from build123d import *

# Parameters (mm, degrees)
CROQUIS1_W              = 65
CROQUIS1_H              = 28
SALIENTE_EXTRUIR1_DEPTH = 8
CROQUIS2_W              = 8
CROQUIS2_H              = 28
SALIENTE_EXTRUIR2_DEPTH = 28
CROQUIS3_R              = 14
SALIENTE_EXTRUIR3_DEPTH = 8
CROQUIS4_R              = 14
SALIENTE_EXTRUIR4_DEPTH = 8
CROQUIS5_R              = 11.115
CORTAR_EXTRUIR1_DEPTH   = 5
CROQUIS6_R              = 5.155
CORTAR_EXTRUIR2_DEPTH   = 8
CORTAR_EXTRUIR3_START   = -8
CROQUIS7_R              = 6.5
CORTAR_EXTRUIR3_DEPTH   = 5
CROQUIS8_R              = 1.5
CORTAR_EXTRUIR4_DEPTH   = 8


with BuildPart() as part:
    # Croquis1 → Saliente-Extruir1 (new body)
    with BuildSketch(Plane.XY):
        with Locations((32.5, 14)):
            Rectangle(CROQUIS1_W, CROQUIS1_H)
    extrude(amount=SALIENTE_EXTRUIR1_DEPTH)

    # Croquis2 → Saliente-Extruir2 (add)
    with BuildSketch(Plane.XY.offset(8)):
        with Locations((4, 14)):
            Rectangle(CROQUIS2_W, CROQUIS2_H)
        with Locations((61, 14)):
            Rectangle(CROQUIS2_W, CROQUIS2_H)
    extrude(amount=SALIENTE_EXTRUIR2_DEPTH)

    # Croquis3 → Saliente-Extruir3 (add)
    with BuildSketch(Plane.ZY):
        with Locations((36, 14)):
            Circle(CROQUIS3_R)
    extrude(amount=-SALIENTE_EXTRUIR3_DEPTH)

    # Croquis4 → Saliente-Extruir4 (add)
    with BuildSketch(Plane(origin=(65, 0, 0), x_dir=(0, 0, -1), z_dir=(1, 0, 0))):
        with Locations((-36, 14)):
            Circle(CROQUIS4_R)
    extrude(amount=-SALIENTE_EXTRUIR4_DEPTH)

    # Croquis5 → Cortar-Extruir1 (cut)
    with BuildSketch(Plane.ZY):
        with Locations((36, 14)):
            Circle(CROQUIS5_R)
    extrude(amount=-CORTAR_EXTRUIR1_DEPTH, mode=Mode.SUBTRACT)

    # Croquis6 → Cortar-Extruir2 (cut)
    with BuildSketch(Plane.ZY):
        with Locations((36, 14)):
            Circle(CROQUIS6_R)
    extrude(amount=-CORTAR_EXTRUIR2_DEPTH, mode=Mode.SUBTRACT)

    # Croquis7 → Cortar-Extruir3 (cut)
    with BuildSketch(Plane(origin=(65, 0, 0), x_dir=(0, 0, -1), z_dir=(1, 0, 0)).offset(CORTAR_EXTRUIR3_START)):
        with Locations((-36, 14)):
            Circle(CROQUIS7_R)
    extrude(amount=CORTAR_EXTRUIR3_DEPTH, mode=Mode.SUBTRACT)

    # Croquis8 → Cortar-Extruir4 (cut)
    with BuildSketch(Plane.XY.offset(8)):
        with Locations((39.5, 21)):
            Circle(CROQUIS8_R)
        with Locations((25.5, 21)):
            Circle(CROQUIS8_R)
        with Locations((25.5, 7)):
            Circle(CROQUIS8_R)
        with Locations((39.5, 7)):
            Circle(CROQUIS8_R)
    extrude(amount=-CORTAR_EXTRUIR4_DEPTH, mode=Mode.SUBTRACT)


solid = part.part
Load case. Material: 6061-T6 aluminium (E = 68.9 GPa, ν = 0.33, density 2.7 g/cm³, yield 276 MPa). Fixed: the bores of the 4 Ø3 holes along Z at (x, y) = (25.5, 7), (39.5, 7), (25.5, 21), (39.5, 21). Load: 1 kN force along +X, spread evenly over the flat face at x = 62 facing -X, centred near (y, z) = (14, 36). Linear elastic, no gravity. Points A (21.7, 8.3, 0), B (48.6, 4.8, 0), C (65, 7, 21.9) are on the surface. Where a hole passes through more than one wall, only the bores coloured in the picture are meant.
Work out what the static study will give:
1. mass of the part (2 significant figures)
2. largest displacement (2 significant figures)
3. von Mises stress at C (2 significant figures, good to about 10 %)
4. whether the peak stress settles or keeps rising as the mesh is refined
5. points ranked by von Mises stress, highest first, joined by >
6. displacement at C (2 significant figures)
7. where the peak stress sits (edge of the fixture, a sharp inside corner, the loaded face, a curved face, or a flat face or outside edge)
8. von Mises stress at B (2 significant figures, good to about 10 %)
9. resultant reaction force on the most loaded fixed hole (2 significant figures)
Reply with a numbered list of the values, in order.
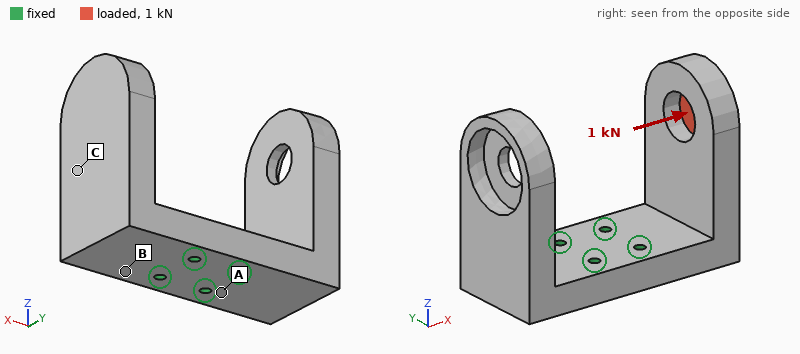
1. 78 g
2. 0.58 mm
3. 47 MPa
4. keeps rising
5. B > C > A
6. 0.23 mm
7. edge of the fixture
8. 99 MPa
9. 550 N
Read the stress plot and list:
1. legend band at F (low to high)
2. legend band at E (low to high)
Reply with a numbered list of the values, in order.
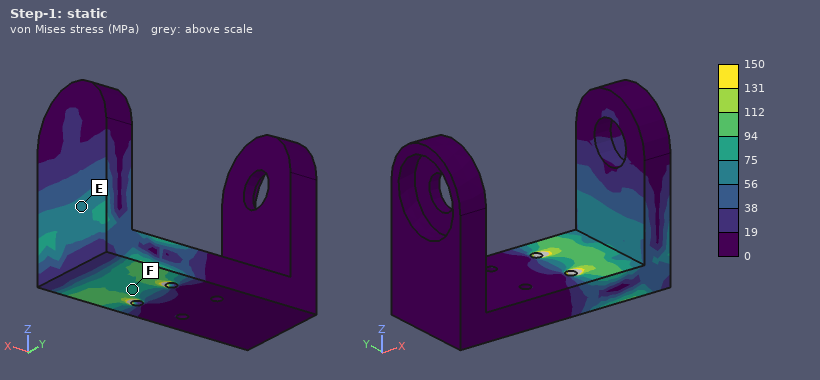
1. 75 to 94 MPa
2. 56 to 75 MPa
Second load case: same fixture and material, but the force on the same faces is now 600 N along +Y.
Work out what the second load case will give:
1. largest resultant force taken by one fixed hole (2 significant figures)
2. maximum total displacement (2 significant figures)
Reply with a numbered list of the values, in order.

1. 1.2 kN
2. 0.13 mm
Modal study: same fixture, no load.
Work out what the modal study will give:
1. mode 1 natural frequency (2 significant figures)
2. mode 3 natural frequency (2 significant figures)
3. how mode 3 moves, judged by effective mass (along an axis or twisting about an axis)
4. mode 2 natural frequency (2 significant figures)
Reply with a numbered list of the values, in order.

1. 2100 Hz
2. 3200 Hz
3. along Y
4. 2400 Hz
